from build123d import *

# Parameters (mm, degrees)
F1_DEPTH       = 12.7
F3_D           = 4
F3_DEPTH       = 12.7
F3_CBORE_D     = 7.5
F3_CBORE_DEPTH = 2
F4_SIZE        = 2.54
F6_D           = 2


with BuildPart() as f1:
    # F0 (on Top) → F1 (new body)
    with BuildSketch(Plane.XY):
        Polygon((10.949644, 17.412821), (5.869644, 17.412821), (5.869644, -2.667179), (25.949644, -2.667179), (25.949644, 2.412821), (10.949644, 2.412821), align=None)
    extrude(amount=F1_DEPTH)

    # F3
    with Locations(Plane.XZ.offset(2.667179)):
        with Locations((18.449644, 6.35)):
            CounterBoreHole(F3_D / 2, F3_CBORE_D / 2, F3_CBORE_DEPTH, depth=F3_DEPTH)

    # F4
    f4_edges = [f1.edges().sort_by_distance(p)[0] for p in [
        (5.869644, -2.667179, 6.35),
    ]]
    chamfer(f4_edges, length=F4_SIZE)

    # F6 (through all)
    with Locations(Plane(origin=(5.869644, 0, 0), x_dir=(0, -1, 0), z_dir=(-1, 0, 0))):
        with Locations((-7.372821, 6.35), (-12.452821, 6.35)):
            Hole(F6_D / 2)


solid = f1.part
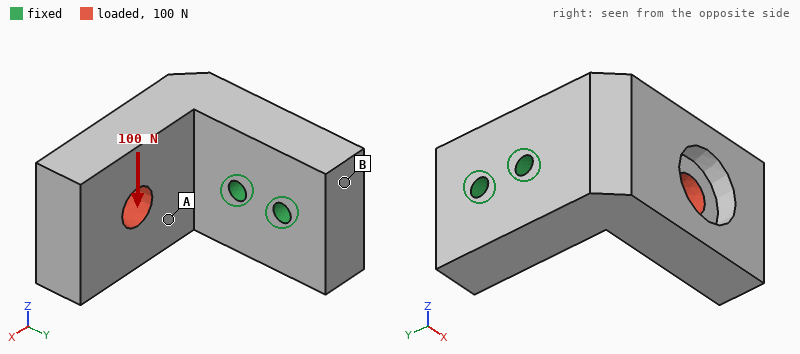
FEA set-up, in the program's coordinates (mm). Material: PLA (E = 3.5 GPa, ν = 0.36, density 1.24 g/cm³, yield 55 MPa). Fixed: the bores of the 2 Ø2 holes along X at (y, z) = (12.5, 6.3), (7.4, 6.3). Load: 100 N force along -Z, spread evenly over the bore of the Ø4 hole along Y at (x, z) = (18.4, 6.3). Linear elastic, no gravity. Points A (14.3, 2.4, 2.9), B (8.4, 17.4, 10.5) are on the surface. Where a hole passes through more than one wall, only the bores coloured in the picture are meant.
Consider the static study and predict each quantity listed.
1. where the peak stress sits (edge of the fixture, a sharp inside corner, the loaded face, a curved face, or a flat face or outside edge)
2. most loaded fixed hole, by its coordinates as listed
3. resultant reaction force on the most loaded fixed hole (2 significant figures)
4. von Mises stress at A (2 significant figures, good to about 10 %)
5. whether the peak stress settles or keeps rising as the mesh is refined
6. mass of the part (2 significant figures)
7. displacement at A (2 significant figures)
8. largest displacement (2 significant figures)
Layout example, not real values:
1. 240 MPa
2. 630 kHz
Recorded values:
1. edge of the fixture
2. (7.4, 6.3)
3. 180 N
4. 6.2 MPa
5. keeps rising
6. 2.6 g
7. 0.11 mm
8. 0.29 mm
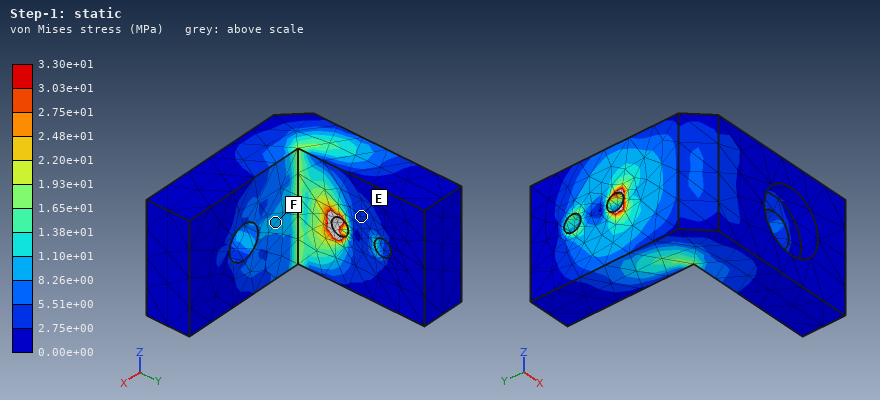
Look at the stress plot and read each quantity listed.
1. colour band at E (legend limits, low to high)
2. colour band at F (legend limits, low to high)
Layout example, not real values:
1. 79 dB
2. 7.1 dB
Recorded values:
1. 2.75e+00 to 5.51e+00 MPa
2. 8.26e+00 to 1.10e+01 MPa
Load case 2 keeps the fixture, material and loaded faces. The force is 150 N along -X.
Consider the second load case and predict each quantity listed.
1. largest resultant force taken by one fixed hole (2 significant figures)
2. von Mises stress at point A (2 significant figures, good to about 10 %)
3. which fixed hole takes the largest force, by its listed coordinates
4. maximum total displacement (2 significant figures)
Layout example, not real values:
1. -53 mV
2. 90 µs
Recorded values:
1. 190 N
2. 5.2 MPa
3. (7.4, 6.3)
4. 0.15 mm
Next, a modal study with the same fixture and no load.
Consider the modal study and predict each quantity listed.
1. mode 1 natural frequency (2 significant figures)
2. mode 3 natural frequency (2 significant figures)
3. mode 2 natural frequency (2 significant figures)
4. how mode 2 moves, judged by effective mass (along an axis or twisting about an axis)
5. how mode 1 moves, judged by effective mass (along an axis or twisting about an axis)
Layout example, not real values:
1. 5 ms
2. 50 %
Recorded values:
1. 2700 Hz
2. 7500 Hz
3. 3300 Hz
4. along Z
5. along Y
